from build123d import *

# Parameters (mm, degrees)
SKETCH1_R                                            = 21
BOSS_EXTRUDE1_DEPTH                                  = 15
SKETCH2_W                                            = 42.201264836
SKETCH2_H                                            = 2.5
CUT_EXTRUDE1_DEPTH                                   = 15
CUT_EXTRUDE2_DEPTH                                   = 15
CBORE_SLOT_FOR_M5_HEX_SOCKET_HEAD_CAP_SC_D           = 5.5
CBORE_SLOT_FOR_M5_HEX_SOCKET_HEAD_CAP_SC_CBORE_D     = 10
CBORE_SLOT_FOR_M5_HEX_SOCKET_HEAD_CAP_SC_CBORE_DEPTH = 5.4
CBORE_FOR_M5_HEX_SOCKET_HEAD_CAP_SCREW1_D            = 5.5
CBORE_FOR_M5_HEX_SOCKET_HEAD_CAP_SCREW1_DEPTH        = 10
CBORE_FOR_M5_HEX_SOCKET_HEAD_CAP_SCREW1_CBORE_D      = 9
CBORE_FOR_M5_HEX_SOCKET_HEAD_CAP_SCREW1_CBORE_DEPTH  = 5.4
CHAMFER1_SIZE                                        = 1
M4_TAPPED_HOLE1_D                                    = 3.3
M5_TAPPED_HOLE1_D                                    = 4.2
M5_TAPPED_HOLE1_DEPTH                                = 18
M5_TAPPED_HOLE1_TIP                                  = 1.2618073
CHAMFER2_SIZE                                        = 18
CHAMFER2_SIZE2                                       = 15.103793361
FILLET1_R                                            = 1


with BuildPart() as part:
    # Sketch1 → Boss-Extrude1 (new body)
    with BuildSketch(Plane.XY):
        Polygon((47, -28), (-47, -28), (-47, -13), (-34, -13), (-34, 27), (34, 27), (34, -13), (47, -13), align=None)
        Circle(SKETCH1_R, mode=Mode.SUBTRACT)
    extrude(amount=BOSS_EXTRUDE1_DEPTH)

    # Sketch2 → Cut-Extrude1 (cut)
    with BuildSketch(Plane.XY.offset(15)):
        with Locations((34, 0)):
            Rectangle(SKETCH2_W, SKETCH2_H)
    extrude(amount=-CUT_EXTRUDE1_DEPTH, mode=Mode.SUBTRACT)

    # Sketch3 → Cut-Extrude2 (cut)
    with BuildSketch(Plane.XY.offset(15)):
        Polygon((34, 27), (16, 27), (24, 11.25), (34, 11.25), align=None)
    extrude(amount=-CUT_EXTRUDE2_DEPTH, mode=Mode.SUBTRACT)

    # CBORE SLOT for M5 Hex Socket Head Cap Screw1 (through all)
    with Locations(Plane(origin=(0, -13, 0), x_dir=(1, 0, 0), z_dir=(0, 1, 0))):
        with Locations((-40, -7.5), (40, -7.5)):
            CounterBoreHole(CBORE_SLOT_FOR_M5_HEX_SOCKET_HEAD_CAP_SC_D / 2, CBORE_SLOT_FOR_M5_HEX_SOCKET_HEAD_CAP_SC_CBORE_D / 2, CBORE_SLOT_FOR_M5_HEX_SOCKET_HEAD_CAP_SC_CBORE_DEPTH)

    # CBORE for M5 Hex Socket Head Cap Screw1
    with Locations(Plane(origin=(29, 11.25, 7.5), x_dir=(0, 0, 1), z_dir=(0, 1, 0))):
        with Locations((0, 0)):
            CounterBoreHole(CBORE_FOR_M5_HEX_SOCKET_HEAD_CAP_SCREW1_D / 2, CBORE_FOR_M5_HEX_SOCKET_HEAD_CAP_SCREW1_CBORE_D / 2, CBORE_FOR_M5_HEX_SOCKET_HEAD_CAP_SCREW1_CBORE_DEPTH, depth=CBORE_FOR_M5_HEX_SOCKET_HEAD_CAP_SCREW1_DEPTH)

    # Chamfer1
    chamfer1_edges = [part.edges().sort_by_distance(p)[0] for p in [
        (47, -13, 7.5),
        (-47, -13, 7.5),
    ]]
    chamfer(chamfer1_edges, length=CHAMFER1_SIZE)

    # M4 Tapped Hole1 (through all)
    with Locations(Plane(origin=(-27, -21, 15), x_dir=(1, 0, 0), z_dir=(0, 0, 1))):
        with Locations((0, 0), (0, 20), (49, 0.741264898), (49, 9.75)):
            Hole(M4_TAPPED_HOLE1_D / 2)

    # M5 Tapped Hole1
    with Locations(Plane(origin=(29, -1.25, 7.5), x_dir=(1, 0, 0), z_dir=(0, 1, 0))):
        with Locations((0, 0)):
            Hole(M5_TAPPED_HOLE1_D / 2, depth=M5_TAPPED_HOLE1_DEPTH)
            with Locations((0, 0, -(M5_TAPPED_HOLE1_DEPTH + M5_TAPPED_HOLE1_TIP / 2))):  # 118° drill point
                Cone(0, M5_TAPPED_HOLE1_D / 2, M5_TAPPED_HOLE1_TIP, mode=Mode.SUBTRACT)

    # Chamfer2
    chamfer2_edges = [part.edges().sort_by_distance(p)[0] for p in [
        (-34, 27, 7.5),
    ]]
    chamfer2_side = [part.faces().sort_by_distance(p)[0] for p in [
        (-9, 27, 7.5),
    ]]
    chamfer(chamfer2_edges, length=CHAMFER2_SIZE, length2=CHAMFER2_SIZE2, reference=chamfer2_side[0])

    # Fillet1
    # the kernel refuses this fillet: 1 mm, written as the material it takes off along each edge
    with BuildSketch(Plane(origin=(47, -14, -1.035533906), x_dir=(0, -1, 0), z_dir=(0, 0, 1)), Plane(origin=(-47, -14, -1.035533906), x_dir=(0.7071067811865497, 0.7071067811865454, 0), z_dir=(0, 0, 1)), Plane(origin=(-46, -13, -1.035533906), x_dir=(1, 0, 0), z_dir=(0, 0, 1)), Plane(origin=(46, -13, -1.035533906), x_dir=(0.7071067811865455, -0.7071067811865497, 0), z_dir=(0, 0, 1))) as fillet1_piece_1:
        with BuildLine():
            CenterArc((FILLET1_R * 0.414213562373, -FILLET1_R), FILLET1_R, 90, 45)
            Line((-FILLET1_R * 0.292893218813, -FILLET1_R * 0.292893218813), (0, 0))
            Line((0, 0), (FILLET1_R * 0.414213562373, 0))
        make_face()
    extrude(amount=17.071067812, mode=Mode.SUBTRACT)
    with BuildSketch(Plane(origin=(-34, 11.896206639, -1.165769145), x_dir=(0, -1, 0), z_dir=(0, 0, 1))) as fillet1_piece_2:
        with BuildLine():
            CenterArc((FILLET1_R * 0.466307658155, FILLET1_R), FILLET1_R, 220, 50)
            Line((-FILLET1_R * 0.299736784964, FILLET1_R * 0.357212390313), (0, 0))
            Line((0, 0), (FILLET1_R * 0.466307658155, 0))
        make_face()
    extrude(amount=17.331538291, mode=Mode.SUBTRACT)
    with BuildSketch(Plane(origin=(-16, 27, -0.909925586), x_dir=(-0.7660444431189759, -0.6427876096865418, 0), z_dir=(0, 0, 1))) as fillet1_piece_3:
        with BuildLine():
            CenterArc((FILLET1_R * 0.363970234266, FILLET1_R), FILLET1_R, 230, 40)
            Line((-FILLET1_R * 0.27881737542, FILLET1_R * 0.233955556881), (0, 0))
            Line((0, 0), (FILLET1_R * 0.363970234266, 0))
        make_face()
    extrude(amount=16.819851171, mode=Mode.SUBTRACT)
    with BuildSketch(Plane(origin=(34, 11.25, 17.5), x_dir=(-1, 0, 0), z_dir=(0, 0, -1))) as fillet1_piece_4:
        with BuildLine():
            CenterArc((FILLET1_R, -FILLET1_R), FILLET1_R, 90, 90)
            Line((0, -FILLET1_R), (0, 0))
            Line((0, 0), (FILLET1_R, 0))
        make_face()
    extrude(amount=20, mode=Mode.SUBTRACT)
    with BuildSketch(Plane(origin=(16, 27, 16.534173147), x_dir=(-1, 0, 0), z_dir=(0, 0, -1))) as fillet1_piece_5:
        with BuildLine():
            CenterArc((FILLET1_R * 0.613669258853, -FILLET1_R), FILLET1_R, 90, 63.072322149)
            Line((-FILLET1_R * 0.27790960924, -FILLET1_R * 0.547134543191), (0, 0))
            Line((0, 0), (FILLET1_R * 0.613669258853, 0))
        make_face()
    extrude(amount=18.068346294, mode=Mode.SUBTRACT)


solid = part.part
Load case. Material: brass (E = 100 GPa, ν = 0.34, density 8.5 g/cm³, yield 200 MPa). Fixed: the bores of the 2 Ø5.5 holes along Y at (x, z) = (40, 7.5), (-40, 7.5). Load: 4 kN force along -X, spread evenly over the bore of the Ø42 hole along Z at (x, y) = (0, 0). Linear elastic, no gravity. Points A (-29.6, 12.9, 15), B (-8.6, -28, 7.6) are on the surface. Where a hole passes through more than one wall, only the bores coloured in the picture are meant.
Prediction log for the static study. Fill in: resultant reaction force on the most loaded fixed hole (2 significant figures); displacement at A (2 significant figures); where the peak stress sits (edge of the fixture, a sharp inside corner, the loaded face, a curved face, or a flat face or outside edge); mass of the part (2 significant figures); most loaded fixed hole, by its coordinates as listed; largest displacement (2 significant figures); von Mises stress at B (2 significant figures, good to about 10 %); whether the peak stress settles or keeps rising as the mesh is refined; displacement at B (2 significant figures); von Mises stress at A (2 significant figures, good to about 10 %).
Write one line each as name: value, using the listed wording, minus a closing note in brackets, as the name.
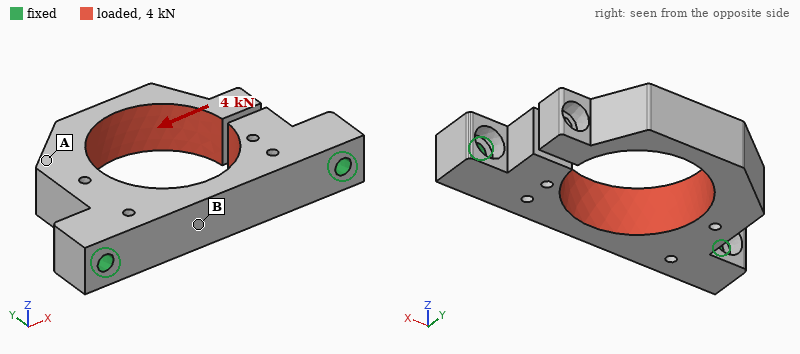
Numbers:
resultant reaction force on the most loaded fixed hole: 3.6 kN
displacement at A: 0.13 mm
where the peak stress sits: edge of the fixture
mass of the part: 280 g
most loaded fixed hole, by its coordinates as listed: (-40, 7.5)
largest displacement: 0.26 mm
von Mises stress at B: 75 MPa
whether the peak stress settles or keeps rising as the mesh is refined: keeps rising
displacement at B: 0.050 mm
von Mises stress at A: 17 MPa
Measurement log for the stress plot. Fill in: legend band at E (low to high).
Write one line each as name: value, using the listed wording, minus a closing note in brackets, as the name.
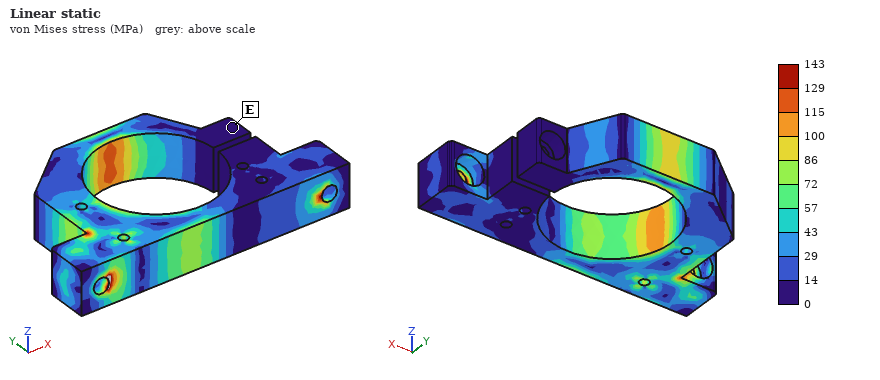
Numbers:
legend band at E: 0 to 14 MPa
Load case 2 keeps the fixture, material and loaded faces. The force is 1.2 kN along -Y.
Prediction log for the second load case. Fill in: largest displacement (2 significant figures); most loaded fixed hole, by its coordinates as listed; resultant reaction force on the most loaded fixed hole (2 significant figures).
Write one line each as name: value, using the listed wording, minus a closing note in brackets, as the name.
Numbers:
largest displacement: 0.31 mm
most loaded fixed hole, by its coordinates as listed: (-40, 7.5)
resultant reaction force on the most loaded fixed hole: 750 N
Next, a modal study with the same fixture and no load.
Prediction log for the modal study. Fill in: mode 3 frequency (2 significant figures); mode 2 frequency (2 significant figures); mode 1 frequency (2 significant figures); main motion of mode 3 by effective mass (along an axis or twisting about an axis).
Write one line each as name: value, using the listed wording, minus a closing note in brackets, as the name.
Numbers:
mode 3 frequency: 1700 Hz
mode 2 frequency: 920 Hz
mode 1 frequency: 910 Hz
main motion of mode 3 by effective mass: along X
